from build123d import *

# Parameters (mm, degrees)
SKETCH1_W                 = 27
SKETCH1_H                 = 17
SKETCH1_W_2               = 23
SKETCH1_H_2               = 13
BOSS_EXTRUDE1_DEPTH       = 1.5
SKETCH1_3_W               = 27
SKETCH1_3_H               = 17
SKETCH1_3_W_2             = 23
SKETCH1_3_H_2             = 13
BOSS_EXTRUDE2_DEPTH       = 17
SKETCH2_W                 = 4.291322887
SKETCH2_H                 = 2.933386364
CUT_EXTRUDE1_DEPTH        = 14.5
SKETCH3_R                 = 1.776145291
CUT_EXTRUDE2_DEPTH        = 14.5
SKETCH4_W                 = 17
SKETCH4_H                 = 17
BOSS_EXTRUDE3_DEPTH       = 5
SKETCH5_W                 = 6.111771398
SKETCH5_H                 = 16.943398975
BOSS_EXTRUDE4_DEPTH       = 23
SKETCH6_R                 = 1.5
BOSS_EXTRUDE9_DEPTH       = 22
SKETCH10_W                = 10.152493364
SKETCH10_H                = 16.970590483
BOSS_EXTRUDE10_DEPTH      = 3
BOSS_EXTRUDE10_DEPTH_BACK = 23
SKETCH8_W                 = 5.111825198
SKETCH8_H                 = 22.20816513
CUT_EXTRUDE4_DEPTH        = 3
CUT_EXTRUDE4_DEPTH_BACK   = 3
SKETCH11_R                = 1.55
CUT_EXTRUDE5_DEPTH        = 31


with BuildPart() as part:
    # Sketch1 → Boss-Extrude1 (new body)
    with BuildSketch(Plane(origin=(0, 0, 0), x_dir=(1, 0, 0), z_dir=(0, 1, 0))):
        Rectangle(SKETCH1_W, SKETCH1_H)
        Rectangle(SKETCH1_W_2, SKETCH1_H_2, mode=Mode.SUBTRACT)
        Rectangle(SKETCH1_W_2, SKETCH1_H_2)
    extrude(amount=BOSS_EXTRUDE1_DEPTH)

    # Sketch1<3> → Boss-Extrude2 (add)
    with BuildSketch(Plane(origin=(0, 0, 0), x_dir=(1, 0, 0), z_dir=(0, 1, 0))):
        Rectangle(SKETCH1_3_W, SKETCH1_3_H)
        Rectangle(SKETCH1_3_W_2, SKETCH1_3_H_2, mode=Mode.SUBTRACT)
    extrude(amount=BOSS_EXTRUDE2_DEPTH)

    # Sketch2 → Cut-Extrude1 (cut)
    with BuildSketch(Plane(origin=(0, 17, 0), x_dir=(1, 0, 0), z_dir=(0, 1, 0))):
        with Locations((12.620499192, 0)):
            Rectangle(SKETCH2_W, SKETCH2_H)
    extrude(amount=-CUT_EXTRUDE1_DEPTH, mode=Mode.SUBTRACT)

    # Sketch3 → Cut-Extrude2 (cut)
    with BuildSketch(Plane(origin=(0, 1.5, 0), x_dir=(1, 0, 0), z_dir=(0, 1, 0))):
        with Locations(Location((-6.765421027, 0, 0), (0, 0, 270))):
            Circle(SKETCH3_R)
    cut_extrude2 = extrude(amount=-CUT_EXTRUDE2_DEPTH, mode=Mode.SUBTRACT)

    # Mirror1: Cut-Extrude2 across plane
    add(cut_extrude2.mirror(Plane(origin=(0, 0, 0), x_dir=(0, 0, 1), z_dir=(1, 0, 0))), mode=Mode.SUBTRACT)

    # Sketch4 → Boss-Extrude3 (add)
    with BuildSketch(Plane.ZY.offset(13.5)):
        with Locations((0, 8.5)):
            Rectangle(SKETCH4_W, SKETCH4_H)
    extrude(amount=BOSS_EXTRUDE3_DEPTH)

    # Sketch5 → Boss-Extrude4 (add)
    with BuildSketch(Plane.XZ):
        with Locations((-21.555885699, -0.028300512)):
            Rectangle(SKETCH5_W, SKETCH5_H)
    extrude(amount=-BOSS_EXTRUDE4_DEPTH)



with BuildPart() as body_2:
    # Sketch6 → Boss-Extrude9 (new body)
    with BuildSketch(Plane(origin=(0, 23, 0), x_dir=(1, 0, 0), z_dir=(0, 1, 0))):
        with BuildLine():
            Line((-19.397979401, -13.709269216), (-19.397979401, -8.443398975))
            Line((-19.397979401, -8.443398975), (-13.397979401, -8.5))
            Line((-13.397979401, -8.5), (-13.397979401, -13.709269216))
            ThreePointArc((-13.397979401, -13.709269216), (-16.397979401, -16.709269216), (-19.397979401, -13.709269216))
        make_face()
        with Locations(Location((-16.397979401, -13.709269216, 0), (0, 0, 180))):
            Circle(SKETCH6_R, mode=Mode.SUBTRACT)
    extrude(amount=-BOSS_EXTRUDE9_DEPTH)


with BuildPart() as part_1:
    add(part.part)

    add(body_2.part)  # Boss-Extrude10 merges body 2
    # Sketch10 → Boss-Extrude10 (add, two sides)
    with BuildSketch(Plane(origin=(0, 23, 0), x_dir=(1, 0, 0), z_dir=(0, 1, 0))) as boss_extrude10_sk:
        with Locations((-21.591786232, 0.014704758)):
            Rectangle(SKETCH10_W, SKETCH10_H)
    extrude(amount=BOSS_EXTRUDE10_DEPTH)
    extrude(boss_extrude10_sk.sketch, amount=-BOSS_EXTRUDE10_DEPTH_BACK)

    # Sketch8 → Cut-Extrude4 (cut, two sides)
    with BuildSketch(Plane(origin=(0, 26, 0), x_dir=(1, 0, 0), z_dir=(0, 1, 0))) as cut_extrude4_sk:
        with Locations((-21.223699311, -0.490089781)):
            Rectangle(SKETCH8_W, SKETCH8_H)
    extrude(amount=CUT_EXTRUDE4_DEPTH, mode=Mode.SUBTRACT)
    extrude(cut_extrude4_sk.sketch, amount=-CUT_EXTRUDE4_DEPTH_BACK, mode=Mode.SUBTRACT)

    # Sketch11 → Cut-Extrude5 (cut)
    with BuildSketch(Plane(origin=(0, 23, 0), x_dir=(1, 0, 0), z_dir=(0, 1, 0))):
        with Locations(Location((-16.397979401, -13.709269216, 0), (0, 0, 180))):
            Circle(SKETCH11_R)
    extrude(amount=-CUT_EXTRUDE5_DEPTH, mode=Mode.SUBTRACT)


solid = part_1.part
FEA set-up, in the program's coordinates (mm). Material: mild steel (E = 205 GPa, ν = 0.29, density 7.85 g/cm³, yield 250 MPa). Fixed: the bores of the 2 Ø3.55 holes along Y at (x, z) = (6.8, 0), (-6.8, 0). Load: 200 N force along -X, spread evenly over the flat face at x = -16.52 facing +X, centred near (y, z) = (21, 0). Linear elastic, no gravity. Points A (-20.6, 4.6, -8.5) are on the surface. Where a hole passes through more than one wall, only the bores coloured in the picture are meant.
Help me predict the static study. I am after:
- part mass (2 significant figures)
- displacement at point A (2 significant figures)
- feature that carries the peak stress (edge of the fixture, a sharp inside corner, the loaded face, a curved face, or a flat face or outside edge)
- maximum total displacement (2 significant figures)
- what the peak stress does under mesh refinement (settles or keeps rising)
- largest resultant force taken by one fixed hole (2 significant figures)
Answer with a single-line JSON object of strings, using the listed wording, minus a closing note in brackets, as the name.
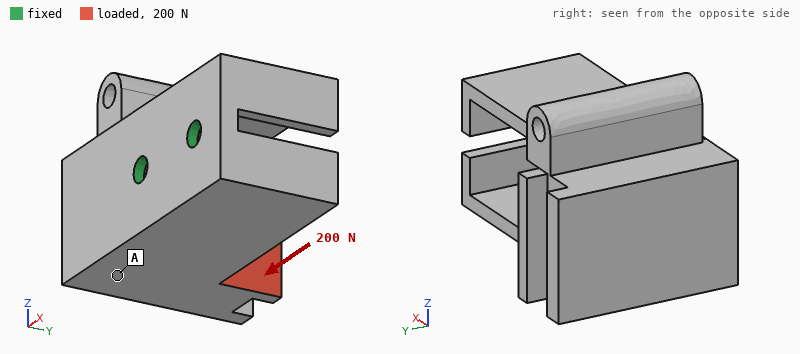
{"part mass": "70 g", "displacement at point A": "9.9 µm", "feature that carries the peak stress": "edge of the fixture", "maximum total displacement": "21 µm", "what the peak stress does under mesh refinement": "keeps rising", "largest resultant force taken by one fixed hole": "260 N"}
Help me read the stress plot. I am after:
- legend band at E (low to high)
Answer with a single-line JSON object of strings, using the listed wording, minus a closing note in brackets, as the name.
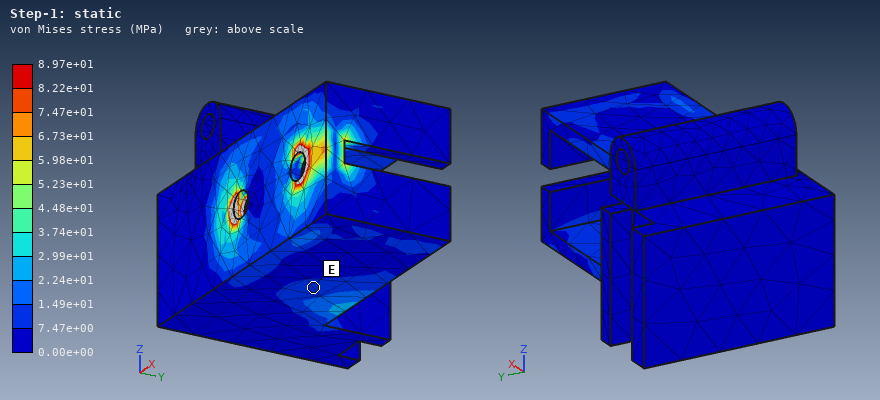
{"legend band at E": "7.47e+00 to 1.49e+01 MPa"}
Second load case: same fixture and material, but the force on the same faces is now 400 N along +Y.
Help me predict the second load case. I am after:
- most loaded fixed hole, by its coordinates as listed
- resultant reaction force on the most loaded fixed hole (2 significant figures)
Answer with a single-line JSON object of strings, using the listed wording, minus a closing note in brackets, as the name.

{"most loaded fixed hole, by its coordinates as listed": "(-6.8, 0)", "resultant reaction force on the most loaded fixed hole": "570 N"}
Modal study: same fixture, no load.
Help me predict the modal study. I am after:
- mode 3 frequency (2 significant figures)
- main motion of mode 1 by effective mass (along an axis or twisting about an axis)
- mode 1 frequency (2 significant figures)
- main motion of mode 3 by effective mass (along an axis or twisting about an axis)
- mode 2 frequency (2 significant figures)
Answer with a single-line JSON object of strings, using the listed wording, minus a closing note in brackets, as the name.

{"mode 3 frequency": "6600 Hz", "main motion of mode 1 by effective mass": "along Z", "mode 1 frequency": "1900 Hz", "main motion of mode 3 by effective mass": "along Y", "mode 2 frequency": "2700 Hz"}
